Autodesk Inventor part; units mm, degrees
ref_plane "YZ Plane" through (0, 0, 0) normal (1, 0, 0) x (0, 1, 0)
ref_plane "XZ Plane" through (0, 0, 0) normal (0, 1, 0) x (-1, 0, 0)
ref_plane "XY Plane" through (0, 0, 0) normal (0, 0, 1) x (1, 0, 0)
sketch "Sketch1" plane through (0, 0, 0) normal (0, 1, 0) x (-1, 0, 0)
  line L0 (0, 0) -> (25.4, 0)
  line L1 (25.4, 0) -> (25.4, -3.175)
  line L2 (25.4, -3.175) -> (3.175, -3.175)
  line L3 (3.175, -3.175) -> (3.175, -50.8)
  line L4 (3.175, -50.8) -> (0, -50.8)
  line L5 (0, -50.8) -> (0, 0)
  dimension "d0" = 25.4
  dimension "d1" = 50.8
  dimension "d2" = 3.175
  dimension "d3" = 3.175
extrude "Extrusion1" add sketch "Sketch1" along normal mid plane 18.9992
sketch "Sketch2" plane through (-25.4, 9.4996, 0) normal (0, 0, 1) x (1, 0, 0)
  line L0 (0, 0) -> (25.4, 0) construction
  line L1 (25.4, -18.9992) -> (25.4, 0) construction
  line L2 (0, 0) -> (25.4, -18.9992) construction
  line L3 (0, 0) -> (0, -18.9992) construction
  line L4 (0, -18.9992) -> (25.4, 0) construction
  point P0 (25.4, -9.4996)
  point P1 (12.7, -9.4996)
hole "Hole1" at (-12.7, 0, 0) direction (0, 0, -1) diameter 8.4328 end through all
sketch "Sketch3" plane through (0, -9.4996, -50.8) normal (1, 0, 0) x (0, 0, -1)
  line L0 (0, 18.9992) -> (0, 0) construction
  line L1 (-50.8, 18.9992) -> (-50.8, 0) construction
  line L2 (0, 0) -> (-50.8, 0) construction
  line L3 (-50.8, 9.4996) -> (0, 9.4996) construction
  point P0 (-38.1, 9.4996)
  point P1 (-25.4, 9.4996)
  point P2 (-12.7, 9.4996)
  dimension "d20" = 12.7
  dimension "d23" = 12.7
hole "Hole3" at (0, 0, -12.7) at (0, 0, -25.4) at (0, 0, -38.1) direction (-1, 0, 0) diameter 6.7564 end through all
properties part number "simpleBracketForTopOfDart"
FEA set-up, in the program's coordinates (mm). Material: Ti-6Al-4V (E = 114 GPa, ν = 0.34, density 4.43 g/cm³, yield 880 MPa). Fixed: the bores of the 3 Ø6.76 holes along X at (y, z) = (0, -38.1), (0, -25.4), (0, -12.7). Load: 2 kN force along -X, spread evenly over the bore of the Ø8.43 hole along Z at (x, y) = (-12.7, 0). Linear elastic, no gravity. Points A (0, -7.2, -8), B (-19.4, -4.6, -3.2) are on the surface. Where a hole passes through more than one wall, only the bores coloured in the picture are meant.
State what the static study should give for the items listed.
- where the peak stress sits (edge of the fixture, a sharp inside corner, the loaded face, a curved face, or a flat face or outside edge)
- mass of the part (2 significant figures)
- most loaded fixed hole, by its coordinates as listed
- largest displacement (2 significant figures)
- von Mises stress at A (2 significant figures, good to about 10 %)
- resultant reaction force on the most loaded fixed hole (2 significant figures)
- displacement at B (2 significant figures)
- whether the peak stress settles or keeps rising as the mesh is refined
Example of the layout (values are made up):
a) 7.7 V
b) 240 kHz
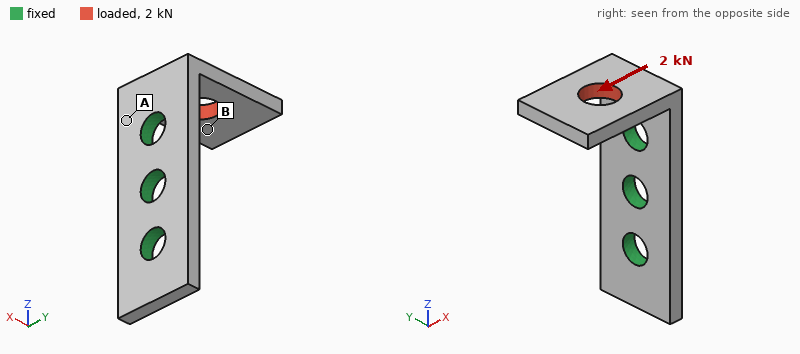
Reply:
a) edge of the fixture
b) 17 g
c) (0, -12.7)
d) 0.35 mm
e) 250 MPa
f) 2.2 kN
g) 0.26 mm
h) keeps rising
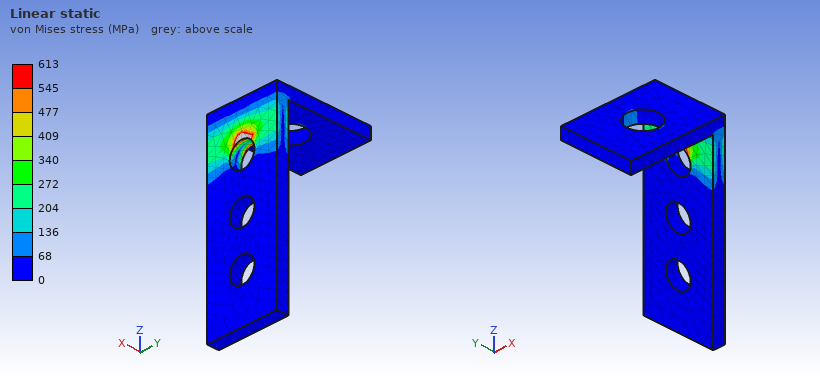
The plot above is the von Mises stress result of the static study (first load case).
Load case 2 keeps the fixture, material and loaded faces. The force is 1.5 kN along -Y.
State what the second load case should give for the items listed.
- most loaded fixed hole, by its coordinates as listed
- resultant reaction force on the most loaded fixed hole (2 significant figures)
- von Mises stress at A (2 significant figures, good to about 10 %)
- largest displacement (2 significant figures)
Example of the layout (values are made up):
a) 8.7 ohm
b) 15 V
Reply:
a) (0, -12.7)
b) 1.9 kN
c) 210 MPa
d) 0.34 mm
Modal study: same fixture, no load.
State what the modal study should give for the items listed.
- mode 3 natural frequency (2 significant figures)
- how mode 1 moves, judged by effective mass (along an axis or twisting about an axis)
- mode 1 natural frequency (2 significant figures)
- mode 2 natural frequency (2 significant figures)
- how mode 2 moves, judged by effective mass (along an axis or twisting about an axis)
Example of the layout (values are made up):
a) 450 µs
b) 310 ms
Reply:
a) 10 kHz
b) along Z
c) 3000 Hz
d) 4900 Hz
e) along Y
